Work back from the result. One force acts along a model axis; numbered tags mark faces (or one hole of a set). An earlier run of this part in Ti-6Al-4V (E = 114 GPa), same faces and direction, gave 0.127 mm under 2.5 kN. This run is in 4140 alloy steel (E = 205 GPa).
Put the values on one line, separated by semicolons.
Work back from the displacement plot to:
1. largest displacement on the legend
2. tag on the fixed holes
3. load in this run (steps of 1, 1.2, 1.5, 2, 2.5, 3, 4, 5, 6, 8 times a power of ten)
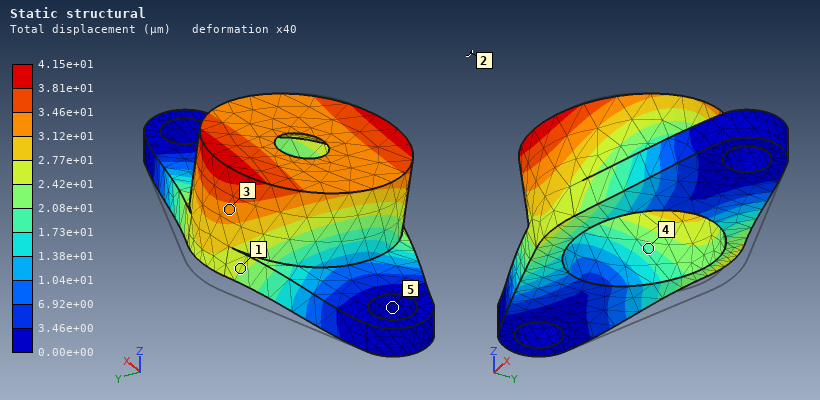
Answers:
4.15e+01 µm; 5; 1.5 kN
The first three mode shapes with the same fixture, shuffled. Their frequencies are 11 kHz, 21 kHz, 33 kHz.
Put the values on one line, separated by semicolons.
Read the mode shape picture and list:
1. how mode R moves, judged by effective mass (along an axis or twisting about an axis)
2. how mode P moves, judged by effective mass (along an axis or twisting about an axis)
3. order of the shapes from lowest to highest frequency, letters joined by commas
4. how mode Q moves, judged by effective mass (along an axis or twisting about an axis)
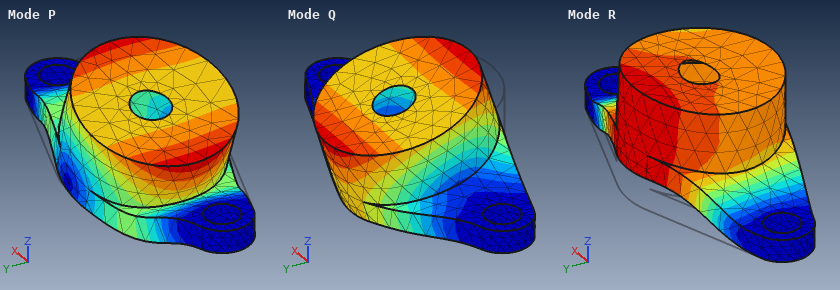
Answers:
along Z; along X; Q, R, P; along Y
